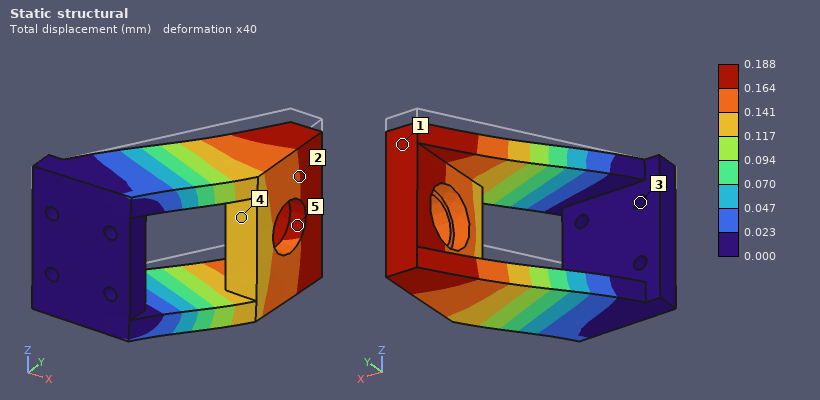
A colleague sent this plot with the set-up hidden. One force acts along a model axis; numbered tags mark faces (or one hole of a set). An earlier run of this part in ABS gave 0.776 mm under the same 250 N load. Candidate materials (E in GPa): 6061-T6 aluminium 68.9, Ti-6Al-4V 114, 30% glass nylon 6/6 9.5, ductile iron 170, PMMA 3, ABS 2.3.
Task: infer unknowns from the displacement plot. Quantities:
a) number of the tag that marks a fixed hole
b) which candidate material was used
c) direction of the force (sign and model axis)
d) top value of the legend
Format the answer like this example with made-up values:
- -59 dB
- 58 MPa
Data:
- 3
- 30% glass nylon 6/6
- -Z
- 0.188 mm
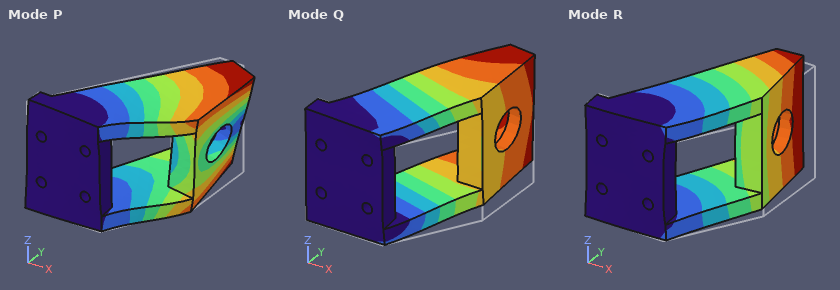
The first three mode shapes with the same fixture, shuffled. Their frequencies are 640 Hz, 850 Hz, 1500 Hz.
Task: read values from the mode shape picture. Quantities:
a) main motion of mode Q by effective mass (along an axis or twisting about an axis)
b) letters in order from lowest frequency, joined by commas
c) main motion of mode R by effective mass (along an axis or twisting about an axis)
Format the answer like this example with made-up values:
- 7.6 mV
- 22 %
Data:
- along Z
- Q, R, P
- along X
